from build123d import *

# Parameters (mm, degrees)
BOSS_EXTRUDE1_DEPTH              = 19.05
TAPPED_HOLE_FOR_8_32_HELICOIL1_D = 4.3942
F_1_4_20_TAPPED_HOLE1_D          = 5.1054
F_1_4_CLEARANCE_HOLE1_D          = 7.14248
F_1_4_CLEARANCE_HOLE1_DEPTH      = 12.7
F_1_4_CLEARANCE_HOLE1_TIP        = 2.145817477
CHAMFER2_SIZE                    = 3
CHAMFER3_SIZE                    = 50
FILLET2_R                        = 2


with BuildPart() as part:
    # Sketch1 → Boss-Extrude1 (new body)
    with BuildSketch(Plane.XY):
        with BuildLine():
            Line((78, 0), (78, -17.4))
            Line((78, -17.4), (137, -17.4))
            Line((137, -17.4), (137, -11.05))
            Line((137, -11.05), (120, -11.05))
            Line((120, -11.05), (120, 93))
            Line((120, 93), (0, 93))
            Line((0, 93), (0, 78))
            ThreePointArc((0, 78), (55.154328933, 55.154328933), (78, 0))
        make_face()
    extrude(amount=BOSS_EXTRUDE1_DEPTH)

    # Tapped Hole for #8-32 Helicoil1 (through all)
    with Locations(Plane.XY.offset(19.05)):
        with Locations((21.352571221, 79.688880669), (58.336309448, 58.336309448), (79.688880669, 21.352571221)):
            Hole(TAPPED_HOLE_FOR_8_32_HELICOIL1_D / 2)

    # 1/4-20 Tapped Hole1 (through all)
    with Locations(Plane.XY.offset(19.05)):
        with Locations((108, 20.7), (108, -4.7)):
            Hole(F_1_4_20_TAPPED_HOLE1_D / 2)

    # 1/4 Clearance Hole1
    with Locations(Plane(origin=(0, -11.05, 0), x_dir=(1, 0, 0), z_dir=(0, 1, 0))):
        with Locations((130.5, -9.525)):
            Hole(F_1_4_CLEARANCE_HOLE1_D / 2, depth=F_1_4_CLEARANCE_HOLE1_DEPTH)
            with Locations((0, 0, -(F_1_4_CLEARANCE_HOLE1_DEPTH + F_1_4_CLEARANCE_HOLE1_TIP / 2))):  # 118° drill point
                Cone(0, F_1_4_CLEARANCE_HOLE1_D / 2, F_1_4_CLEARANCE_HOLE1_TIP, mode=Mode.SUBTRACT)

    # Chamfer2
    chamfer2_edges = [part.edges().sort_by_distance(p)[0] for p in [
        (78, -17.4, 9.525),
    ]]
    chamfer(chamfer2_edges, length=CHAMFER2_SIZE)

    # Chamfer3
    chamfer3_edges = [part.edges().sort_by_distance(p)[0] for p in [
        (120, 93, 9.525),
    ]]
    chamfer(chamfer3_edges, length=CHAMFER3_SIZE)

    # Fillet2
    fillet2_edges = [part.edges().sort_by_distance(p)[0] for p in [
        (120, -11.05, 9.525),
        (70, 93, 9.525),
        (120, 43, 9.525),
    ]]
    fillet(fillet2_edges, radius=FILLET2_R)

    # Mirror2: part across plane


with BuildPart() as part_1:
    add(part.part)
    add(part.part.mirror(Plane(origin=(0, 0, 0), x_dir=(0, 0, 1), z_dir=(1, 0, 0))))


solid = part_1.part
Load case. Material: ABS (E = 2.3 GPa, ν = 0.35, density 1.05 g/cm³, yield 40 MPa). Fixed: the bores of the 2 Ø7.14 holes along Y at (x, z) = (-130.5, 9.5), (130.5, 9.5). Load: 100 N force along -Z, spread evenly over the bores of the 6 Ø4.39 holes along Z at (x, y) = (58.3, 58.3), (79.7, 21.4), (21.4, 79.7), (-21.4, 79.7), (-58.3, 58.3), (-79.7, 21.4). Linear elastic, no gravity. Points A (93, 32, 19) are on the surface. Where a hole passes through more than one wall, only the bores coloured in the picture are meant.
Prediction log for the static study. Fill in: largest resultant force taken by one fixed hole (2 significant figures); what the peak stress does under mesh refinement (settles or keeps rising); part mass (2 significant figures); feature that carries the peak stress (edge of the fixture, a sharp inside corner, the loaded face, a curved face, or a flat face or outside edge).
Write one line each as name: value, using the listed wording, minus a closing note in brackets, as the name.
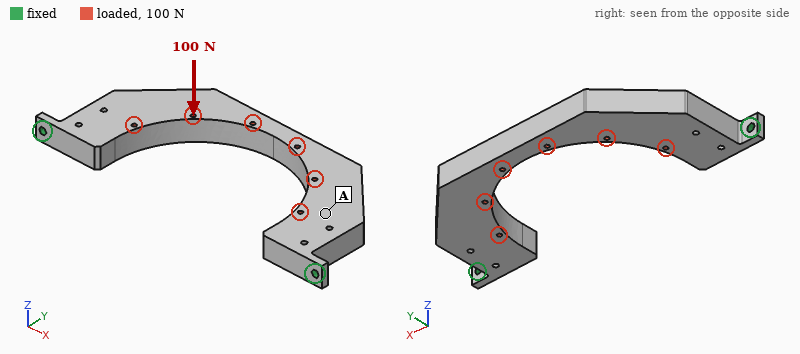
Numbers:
largest resultant force taken by one fixed hole: 50 N
what the peak stress does under mesh refinement: keeps rising
part mass: 230 g
feature that carries the peak stress: edge of the fixture
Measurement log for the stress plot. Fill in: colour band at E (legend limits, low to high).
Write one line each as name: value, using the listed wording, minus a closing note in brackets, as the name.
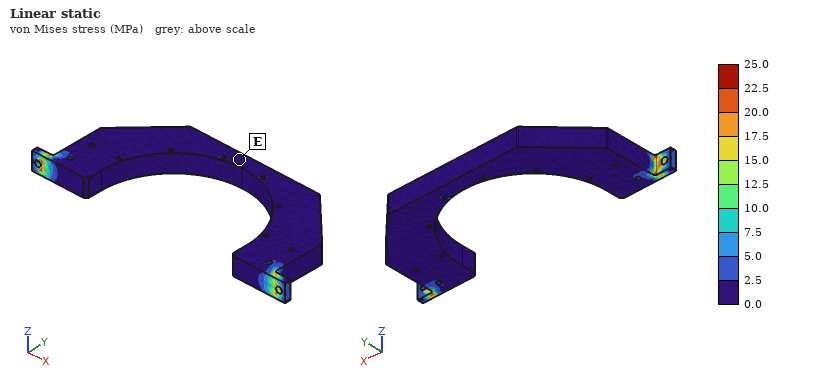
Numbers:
colour band at E: 0.0 to 2.5 MPa
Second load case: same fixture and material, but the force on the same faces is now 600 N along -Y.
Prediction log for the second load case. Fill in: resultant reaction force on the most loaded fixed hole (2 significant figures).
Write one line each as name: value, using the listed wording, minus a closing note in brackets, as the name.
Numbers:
resultant reaction force on the most loaded fixed hole: 360 N
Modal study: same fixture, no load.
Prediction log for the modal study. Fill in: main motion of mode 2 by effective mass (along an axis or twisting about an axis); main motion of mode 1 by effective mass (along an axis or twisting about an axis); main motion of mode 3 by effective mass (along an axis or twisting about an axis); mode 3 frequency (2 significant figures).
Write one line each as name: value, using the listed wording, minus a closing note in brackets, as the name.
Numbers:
main motion of mode 2 by effective mass: twisting about Y
main motion of mode 1 by effective mass: along Z
main motion of mode 3 by effective mass: along X
mode 3 frequency: 470 Hz
